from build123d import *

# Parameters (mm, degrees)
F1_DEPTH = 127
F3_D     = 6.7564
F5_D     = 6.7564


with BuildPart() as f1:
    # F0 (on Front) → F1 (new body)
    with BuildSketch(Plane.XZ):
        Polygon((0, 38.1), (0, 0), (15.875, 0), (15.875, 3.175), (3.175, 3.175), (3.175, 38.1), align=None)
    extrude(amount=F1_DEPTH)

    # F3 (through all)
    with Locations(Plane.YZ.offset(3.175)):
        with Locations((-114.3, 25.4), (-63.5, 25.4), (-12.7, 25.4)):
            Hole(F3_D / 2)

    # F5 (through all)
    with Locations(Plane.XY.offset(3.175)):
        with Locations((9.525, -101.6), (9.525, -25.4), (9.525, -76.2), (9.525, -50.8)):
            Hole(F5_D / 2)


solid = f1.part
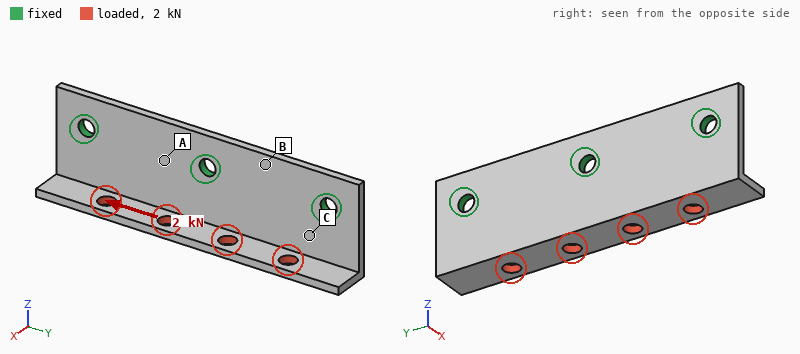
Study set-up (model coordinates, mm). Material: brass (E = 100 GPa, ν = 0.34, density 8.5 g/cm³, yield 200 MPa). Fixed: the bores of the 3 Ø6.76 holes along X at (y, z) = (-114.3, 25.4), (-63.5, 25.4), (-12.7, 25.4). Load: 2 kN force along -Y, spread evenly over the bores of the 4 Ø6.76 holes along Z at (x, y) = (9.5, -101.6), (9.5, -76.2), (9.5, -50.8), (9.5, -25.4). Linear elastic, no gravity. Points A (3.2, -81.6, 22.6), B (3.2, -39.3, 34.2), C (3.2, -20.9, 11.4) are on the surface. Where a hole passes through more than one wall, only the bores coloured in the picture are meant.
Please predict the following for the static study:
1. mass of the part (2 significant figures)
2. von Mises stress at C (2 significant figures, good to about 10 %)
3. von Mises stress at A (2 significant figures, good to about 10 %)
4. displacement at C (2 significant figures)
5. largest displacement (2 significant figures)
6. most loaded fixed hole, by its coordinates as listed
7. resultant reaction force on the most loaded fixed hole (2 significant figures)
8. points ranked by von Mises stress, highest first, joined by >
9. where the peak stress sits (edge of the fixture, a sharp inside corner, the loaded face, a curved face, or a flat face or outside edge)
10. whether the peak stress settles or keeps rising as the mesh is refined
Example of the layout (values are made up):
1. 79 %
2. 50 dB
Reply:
1. 170 g
2. 27 MPa
3. 12 MPa
4. 19 µm
5. 84 µm
6. (-63.5, 25.4)
7. 880 N
8. C > A > B
9. edge of the fixture
10. keeps rising
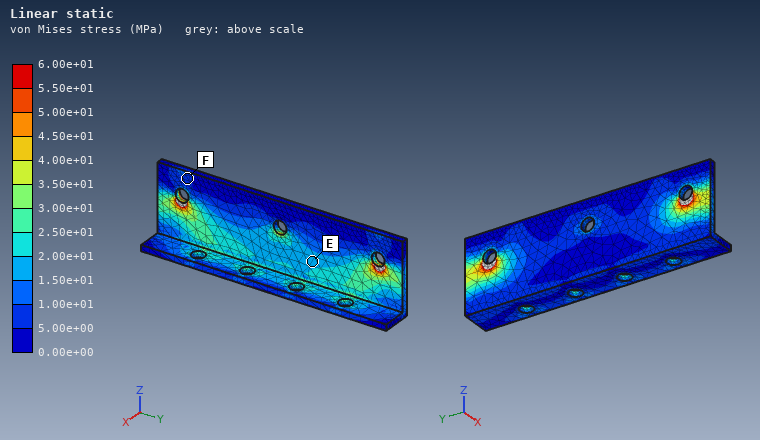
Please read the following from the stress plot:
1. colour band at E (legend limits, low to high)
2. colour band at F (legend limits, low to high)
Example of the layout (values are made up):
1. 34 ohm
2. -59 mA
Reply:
1. 1.50e+01 to 2.00e+01 MPa
2. 5.00e+00 to 1.00e+01 MPa
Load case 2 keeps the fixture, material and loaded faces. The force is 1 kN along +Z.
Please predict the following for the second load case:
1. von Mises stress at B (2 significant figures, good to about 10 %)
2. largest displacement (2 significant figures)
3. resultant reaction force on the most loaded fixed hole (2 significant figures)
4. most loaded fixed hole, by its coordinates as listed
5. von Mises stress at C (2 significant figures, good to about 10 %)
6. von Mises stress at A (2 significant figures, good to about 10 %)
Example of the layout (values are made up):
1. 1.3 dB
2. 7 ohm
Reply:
1. 7.0 MPa
2. 0.12 mm
3. 600 N
4. (-63.5, 25.4)
5. 35 MPa
6. 21 MPa
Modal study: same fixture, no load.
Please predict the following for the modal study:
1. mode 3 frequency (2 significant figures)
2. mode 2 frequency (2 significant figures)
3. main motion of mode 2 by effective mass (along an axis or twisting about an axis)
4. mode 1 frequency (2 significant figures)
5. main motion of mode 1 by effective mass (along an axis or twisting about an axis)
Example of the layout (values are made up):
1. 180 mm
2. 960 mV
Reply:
1. 4200 Hz
2. 1900 Hz
3. twisting about Z
4. 1500 Hz
5. along X
